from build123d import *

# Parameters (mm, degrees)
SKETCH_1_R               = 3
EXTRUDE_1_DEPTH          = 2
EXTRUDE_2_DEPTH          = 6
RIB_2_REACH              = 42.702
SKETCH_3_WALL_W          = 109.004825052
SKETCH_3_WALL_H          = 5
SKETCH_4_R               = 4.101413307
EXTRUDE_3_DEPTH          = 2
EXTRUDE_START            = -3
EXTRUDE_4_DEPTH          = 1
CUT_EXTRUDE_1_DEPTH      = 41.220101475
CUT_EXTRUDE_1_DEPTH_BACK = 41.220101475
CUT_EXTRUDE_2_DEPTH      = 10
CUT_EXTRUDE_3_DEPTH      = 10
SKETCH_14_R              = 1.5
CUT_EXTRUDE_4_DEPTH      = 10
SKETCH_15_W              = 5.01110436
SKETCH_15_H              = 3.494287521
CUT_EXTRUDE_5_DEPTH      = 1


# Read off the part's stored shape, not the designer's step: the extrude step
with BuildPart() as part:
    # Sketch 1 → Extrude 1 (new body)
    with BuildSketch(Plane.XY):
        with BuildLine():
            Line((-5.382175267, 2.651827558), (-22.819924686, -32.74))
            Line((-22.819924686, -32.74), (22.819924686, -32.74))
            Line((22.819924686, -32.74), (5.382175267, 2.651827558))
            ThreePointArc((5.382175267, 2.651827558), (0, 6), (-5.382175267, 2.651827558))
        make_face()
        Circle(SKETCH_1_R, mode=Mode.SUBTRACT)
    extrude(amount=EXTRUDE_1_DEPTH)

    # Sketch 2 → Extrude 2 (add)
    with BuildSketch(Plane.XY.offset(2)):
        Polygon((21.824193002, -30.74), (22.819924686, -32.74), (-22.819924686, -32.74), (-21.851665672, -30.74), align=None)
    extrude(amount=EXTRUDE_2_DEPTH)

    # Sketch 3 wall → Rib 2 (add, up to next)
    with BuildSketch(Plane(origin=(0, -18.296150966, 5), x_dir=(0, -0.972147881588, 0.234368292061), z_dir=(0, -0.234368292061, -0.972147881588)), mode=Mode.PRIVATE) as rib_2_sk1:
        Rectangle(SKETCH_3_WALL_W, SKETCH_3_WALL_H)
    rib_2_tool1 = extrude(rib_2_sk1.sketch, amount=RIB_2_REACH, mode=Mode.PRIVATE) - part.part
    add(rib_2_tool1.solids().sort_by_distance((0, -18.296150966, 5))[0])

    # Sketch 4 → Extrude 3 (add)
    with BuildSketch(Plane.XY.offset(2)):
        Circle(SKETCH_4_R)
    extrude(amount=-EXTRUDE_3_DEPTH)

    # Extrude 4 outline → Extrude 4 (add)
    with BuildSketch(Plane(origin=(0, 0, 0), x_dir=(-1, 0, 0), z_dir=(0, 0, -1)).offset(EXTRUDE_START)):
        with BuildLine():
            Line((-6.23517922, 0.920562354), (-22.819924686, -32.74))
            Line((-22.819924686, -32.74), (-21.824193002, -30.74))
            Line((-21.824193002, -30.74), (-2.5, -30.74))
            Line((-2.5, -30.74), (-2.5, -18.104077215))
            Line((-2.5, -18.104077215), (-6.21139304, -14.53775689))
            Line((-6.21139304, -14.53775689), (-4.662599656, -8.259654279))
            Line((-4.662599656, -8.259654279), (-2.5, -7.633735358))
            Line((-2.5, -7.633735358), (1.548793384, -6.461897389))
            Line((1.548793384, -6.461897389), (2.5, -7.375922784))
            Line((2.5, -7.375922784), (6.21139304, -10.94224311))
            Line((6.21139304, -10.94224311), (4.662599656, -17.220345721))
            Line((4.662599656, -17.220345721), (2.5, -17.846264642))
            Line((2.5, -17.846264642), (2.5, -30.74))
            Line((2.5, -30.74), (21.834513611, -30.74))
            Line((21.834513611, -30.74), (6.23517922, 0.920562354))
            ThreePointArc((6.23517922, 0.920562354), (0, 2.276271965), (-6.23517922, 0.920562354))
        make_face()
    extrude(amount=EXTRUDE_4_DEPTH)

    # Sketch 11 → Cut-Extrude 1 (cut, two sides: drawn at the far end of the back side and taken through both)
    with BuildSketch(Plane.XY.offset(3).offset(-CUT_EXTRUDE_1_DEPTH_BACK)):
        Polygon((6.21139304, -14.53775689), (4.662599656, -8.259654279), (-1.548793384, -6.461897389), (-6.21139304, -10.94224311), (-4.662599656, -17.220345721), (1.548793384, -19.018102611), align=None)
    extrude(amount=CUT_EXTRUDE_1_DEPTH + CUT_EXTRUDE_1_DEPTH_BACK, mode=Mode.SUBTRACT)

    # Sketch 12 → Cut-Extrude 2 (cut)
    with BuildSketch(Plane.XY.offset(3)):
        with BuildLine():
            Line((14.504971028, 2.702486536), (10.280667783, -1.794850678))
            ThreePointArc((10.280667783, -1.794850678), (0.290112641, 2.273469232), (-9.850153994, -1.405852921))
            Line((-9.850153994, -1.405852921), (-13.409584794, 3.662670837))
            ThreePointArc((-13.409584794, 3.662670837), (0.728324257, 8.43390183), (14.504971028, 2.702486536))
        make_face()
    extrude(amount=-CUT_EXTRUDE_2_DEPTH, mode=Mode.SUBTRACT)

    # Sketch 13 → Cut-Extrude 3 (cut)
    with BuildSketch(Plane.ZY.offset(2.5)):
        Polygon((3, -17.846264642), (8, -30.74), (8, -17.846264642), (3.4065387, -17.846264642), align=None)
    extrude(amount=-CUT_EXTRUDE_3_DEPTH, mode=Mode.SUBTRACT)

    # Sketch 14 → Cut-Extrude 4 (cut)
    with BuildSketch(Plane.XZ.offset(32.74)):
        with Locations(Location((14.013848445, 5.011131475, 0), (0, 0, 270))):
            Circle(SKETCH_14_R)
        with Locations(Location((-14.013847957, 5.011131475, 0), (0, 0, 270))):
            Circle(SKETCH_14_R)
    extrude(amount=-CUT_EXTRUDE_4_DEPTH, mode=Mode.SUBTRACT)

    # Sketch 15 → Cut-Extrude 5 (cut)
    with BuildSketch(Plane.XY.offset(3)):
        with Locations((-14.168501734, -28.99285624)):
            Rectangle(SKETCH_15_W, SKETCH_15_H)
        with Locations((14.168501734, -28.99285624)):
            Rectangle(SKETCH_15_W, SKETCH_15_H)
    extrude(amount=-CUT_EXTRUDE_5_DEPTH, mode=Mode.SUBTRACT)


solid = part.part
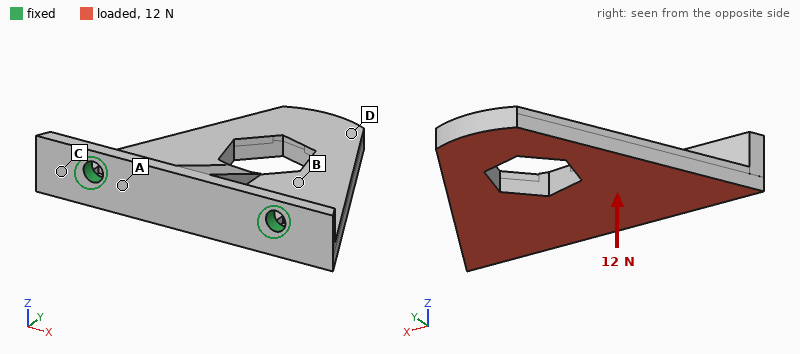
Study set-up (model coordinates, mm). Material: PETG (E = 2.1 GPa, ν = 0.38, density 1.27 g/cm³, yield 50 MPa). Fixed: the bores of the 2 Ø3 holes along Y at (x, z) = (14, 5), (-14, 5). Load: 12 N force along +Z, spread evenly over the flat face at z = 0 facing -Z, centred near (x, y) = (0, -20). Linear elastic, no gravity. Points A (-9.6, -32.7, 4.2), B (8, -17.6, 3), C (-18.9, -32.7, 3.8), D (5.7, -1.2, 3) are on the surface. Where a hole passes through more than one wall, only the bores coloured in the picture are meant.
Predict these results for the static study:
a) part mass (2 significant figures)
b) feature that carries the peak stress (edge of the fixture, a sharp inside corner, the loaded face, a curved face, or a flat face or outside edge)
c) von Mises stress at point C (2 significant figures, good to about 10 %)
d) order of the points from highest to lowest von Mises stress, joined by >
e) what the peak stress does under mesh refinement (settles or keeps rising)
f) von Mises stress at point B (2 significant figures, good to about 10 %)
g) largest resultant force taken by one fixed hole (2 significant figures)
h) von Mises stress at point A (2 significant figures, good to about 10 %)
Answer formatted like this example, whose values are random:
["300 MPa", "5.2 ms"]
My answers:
["4.0 g", "edge of the fixture", "3.0 MPa", "A > C > B > D", "keeps rising", "1.5 MPa", "6.2 N", "3.8 MPa"]
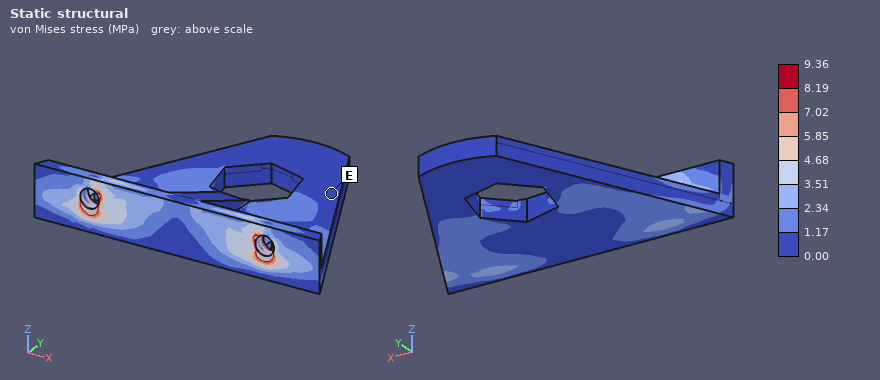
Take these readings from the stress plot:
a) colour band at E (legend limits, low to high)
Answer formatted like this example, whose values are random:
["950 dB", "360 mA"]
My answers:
["0.00 to 1.17 MPa"]
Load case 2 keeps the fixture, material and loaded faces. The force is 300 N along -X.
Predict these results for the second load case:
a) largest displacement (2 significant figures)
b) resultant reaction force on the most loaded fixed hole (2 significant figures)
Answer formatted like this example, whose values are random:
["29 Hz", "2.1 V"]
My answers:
["0.33 mm", "200 N"]
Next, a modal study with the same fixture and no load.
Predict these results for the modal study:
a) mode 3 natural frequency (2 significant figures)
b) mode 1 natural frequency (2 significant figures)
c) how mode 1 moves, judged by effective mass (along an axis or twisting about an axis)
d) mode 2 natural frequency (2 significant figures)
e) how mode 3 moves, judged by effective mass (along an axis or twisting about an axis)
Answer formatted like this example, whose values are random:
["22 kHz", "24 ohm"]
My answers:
["2400 Hz", "510 Hz", "along Z", "2000 Hz", "along Z"]
